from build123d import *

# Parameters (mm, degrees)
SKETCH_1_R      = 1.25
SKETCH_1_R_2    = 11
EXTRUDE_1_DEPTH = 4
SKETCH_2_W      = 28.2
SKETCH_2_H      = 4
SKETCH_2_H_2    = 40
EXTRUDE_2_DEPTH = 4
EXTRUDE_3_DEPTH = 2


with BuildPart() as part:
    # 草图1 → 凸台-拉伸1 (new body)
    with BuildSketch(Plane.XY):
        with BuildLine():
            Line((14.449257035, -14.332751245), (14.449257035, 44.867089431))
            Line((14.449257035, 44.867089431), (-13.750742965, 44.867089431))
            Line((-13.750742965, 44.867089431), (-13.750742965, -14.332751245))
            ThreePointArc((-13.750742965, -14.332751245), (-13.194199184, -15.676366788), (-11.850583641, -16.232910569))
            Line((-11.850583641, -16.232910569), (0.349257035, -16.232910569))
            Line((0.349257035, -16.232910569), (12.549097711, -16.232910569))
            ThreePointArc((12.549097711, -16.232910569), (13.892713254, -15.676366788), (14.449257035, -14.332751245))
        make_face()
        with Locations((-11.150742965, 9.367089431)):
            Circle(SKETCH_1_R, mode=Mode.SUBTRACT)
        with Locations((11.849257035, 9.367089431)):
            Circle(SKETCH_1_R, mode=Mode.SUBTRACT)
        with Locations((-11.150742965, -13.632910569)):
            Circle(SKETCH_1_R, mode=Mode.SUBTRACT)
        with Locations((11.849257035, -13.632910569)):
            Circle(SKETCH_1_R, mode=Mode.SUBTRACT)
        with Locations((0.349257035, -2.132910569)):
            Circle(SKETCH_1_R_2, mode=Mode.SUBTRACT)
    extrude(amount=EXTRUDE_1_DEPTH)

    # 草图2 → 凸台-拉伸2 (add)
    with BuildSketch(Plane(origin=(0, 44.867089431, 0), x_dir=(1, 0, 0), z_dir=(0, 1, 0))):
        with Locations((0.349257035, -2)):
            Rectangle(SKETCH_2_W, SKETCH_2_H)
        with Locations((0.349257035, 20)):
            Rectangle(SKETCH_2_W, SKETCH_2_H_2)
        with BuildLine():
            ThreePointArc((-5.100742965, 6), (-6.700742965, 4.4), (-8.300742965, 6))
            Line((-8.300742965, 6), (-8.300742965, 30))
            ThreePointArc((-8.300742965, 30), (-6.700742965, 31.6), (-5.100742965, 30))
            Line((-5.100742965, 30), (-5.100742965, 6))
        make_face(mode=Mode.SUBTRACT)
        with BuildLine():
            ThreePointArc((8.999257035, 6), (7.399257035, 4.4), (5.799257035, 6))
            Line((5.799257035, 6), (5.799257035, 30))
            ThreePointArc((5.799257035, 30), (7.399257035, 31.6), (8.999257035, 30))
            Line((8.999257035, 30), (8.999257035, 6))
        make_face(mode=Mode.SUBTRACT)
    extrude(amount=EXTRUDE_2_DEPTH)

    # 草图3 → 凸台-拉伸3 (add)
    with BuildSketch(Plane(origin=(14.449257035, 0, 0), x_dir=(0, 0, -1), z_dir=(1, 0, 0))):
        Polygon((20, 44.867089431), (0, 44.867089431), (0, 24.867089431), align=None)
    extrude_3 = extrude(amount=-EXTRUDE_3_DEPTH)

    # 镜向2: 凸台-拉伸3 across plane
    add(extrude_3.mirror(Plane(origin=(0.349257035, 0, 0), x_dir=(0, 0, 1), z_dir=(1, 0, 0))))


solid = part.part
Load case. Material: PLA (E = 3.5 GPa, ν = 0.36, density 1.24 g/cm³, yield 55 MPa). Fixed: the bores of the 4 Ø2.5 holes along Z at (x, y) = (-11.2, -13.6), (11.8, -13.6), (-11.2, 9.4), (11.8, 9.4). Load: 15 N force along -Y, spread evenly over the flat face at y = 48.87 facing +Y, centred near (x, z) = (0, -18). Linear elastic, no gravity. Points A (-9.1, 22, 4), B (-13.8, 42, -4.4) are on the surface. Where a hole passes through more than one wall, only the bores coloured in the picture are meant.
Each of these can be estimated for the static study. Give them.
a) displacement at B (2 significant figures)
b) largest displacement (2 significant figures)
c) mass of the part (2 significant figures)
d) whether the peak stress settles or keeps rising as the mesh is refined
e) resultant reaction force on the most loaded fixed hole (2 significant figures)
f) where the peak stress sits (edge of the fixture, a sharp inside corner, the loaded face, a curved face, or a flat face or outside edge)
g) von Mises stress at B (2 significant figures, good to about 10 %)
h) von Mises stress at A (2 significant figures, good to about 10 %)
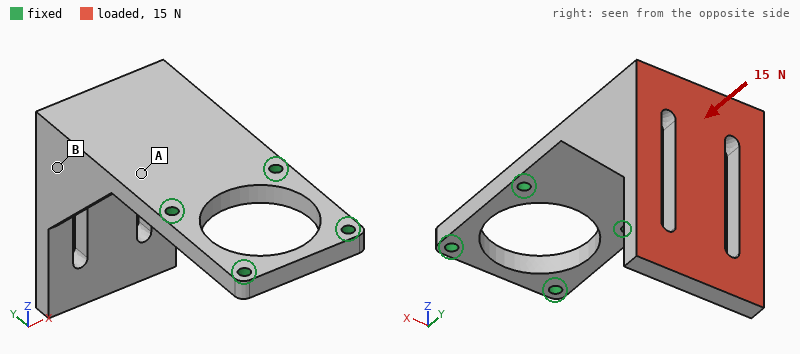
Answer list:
0.33 mm
0.81 mm
13 g
keeps rising
7.6 N
edge of the fixture
0.74 MPa
4.1 MPa
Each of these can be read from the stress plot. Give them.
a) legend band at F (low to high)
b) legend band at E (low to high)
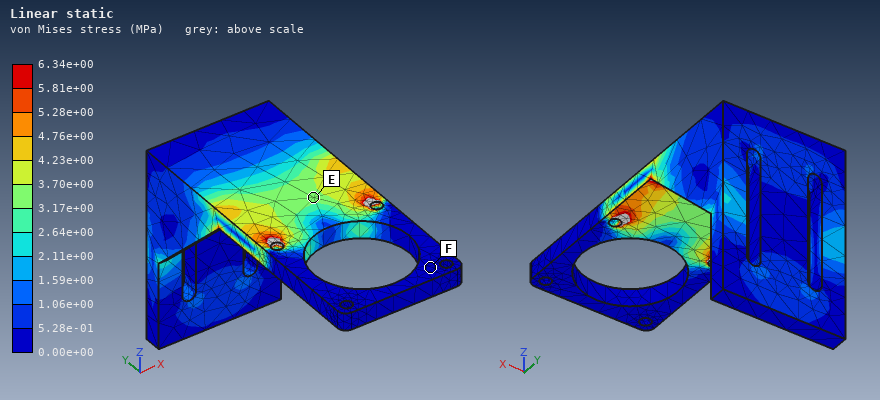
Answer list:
0.00e+00 to 5.28e-01 MPa
3.17e+00 to 3.70e+00 MPa
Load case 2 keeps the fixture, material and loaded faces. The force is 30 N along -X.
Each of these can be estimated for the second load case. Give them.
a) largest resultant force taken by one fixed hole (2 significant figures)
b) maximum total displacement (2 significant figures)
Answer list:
59 N
0.78 mm
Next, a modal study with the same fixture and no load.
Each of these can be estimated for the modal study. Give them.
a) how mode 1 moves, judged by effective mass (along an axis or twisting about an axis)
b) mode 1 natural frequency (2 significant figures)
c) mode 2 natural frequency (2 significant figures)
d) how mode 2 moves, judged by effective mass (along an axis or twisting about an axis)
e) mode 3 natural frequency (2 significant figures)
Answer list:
along Z
250 Hz
480 Hz
along X
1100 Hz
